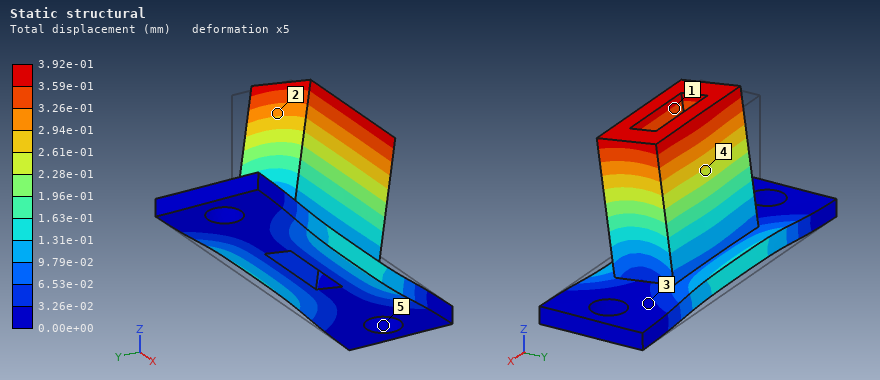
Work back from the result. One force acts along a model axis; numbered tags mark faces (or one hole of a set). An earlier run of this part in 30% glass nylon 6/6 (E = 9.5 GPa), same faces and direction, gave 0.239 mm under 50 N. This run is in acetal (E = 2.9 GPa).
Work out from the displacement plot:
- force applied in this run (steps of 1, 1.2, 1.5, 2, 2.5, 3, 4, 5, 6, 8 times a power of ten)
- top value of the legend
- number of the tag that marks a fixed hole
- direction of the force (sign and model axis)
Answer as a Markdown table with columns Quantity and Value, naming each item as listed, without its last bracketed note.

| Quantity | Value |
|---|---|
| force applied in this run | 25 N |
| top value of the legend | 3.92e-01 mm |
| number of the tag that marks a fixed hole | 5 |
| direction of the force | -Y |
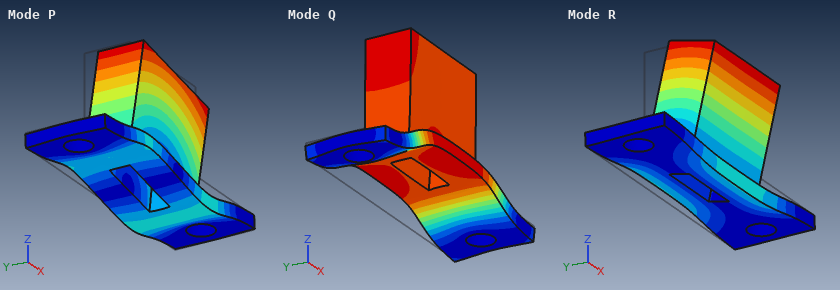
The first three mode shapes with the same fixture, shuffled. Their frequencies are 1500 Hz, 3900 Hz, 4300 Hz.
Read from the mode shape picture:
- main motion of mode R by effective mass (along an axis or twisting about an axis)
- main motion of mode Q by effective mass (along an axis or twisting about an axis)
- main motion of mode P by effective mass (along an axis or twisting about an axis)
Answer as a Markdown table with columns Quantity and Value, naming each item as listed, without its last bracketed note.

| Quantity | Value |
|---|---|
| main motion of mode R by effective mass | along Y |
| main motion of mode Q by effective mass | along Z |
| main motion of mode P by effective mass | along X |
